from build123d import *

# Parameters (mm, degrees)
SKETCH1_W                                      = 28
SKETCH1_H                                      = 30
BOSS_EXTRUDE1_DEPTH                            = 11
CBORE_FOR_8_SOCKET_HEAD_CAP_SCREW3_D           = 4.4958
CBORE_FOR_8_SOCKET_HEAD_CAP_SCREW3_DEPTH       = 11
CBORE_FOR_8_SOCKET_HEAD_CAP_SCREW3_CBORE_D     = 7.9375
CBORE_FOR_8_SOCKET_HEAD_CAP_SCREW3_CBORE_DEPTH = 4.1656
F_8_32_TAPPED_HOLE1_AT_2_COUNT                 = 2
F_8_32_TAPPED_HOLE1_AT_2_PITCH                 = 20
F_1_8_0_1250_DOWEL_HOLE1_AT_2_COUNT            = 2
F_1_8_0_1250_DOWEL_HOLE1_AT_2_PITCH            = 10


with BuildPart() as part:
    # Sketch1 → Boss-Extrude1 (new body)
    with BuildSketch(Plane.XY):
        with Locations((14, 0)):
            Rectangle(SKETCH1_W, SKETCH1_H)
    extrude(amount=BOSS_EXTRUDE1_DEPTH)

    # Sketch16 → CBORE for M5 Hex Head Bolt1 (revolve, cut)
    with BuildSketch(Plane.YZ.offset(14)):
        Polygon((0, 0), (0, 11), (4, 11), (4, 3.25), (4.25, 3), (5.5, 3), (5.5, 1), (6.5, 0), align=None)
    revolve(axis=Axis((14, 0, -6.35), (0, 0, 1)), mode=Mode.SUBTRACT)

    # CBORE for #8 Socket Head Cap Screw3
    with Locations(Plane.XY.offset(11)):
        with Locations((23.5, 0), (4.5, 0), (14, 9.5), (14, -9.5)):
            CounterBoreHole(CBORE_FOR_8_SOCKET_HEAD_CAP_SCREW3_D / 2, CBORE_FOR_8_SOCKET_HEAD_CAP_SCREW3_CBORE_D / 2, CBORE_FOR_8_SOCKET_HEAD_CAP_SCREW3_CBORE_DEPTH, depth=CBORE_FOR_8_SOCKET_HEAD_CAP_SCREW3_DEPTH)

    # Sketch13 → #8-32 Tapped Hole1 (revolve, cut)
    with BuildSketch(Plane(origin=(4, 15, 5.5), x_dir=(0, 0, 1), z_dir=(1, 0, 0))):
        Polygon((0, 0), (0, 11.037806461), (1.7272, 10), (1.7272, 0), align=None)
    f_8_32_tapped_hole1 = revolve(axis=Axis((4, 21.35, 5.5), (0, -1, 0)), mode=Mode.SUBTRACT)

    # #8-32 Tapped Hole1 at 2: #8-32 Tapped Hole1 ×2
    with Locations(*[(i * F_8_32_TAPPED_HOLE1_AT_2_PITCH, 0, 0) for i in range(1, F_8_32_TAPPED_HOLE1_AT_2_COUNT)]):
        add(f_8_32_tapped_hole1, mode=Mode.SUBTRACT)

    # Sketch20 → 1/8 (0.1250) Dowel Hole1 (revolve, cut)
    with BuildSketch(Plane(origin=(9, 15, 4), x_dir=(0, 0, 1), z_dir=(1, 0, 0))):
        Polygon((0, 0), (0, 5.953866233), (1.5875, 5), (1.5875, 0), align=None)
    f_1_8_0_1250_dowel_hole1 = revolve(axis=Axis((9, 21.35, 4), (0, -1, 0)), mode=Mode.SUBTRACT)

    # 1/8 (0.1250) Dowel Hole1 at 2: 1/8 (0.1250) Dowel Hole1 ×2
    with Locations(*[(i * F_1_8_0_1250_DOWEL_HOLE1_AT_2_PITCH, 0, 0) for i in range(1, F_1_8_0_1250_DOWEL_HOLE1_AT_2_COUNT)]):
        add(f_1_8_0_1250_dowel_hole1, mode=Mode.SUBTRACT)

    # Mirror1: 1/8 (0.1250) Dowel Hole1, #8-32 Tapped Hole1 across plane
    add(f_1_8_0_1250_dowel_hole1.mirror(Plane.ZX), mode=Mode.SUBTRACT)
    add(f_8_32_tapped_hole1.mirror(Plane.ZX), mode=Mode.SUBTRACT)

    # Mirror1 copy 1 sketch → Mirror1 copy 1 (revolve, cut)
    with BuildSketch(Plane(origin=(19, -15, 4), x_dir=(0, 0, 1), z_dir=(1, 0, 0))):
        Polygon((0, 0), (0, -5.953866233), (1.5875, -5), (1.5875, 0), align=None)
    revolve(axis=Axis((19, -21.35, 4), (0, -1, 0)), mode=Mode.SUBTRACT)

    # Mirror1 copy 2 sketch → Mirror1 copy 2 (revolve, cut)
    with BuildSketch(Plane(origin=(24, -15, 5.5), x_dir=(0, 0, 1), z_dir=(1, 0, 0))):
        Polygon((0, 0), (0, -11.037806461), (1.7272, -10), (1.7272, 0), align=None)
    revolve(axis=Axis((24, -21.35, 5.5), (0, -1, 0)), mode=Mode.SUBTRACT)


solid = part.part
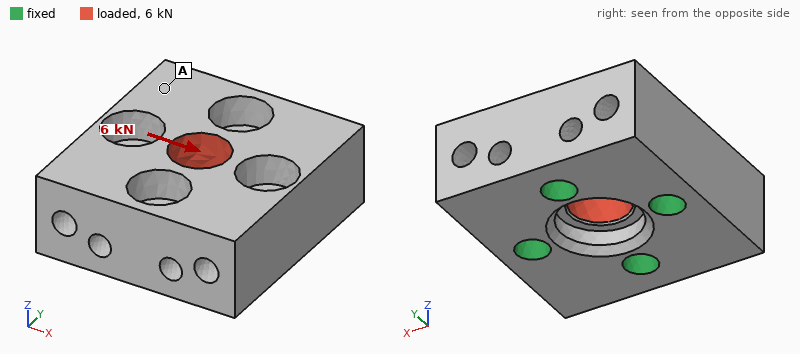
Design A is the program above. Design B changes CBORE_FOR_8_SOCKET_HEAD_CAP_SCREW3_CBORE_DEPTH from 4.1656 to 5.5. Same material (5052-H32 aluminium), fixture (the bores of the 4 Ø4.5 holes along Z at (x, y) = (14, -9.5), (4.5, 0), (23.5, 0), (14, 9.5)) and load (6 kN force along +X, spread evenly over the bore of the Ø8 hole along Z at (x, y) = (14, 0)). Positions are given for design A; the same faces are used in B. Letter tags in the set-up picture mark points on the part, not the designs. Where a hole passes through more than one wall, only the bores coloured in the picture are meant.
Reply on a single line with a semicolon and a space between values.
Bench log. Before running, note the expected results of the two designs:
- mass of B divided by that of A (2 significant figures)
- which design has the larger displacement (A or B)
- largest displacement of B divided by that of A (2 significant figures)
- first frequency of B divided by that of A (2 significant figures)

0.97; B; 1.3; 0.87
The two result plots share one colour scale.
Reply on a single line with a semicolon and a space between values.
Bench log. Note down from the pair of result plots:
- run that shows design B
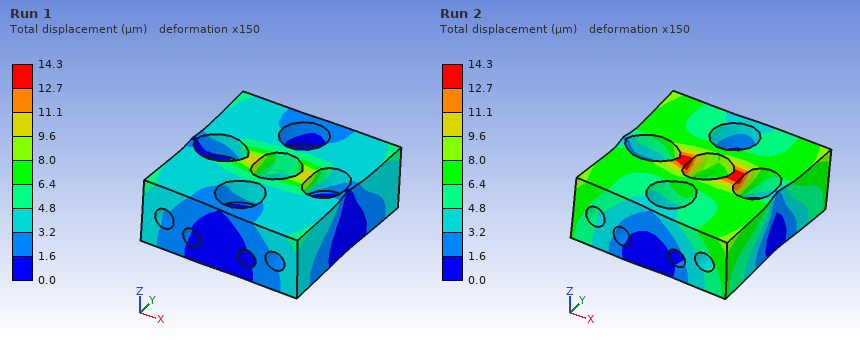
Run 2
